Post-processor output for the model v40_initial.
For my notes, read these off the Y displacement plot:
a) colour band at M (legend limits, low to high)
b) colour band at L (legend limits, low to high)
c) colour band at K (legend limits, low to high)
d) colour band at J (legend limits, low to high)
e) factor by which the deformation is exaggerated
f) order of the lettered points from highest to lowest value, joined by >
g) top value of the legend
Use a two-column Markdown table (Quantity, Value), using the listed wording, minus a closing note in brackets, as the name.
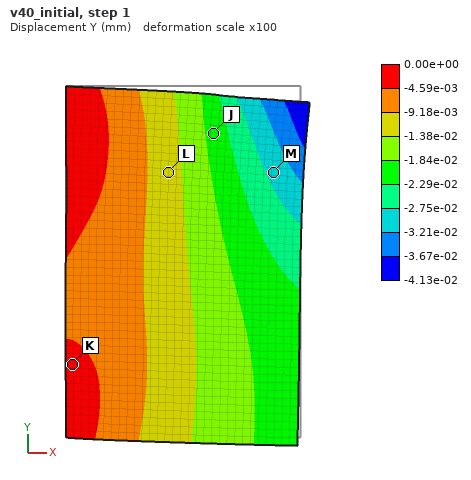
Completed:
| Quantity | Value |
|---|---|
| colour band at M | -3.21e-02 to -2.75e-02 mm |
| colour band at L | -1.38e-02 to -9.18e-03 mm |
| colour band at K | -4.59e-03 to 0.00e+00 mm |
| colour band at J | -2.29e-02 to -1.84e-02 mm |
| factor by which the deformation is exaggerated | 100 |
| order of the lettered points from highest to lowest value, joined by > | K > L > J > M |
| top value of the legend | 0.00e+00 mm |
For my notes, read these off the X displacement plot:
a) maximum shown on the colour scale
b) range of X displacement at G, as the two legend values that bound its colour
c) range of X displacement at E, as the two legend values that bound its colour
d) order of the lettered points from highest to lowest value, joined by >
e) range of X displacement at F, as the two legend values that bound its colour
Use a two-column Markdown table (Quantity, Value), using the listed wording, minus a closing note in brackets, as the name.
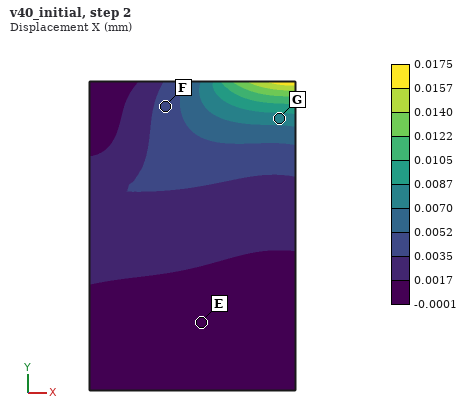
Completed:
| Quantity | Value |
|---|---|
| maximum shown on the colour scale | 0.0175 mm |
| range of X displacement at G, as the two legend values that bound its colour | 0.0070 to 0.0087 mm |
| range of X displacement at E, as the two legend values that bound its colour | -0.0001 to 0.0017 mm |
| order of the lettered points from highest to lowest value, joined by > | G > F > E |
| range of X displacement at F, as the two legend values that bound its colour | 0.0035 to 0.0052 mm |
